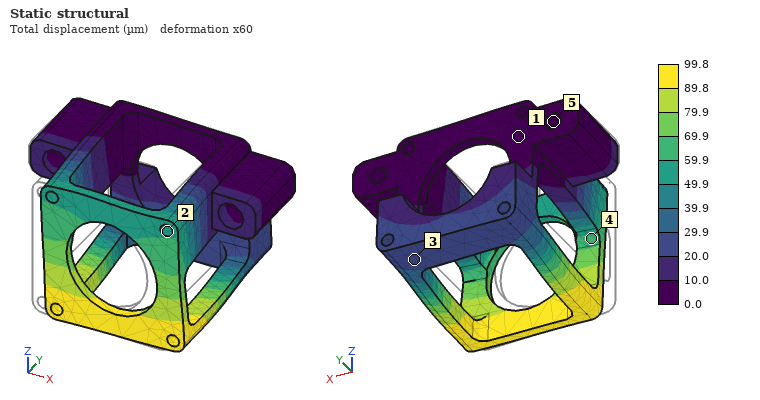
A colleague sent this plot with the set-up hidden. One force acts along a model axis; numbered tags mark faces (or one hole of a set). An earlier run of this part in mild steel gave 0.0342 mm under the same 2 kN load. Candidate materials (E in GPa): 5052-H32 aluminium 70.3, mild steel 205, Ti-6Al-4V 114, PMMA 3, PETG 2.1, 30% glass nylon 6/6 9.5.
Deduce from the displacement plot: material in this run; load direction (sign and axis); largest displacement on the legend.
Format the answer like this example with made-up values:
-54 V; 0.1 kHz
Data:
5052-H32 aluminium; +X; 99.8 µm
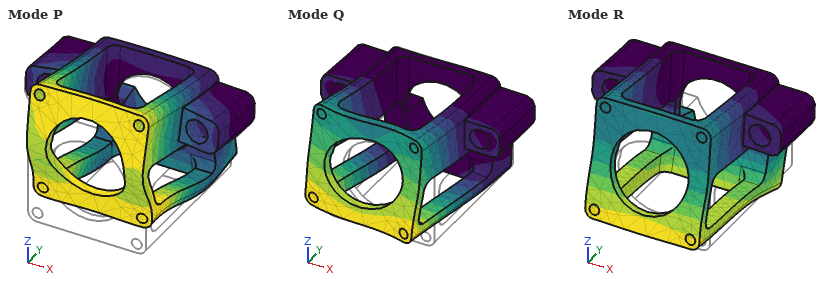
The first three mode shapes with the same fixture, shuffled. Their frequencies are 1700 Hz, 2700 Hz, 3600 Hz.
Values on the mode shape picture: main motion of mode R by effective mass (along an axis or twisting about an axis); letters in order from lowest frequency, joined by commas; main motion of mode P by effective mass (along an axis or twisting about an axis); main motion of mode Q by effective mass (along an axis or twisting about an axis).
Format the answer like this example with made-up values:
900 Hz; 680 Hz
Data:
along Y; R, Q, P; along Z; along X
